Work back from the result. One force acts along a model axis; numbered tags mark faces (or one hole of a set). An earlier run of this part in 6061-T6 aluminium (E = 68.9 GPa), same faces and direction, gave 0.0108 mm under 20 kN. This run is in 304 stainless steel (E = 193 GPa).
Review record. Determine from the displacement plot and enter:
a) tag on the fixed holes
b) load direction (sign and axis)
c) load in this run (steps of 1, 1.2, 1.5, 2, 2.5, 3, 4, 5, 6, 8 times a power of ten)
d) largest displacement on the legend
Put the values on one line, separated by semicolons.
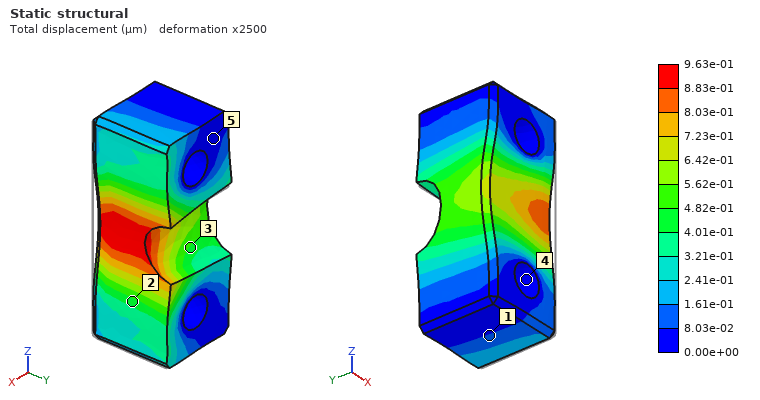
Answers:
4; -X; 5 kN; 9.63e-01 µm
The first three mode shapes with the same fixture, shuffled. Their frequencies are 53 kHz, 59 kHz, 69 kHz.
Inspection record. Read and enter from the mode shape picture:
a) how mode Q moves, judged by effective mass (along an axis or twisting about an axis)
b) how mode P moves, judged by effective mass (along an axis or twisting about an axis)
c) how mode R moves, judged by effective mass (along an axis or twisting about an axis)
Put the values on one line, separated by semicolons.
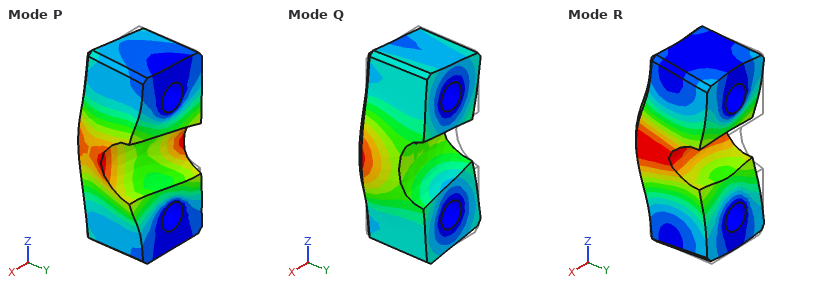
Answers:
along X; twisting about Z; along Y
